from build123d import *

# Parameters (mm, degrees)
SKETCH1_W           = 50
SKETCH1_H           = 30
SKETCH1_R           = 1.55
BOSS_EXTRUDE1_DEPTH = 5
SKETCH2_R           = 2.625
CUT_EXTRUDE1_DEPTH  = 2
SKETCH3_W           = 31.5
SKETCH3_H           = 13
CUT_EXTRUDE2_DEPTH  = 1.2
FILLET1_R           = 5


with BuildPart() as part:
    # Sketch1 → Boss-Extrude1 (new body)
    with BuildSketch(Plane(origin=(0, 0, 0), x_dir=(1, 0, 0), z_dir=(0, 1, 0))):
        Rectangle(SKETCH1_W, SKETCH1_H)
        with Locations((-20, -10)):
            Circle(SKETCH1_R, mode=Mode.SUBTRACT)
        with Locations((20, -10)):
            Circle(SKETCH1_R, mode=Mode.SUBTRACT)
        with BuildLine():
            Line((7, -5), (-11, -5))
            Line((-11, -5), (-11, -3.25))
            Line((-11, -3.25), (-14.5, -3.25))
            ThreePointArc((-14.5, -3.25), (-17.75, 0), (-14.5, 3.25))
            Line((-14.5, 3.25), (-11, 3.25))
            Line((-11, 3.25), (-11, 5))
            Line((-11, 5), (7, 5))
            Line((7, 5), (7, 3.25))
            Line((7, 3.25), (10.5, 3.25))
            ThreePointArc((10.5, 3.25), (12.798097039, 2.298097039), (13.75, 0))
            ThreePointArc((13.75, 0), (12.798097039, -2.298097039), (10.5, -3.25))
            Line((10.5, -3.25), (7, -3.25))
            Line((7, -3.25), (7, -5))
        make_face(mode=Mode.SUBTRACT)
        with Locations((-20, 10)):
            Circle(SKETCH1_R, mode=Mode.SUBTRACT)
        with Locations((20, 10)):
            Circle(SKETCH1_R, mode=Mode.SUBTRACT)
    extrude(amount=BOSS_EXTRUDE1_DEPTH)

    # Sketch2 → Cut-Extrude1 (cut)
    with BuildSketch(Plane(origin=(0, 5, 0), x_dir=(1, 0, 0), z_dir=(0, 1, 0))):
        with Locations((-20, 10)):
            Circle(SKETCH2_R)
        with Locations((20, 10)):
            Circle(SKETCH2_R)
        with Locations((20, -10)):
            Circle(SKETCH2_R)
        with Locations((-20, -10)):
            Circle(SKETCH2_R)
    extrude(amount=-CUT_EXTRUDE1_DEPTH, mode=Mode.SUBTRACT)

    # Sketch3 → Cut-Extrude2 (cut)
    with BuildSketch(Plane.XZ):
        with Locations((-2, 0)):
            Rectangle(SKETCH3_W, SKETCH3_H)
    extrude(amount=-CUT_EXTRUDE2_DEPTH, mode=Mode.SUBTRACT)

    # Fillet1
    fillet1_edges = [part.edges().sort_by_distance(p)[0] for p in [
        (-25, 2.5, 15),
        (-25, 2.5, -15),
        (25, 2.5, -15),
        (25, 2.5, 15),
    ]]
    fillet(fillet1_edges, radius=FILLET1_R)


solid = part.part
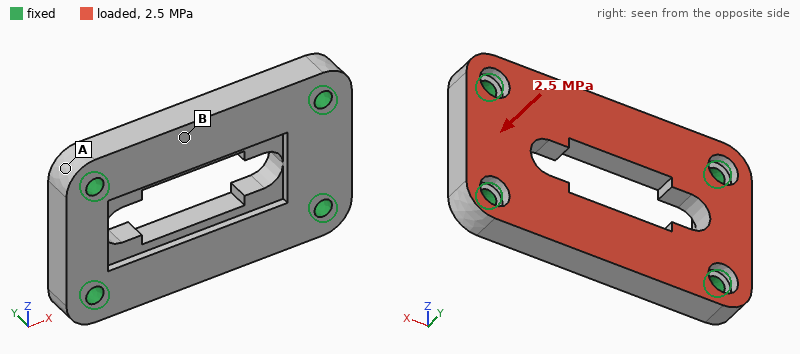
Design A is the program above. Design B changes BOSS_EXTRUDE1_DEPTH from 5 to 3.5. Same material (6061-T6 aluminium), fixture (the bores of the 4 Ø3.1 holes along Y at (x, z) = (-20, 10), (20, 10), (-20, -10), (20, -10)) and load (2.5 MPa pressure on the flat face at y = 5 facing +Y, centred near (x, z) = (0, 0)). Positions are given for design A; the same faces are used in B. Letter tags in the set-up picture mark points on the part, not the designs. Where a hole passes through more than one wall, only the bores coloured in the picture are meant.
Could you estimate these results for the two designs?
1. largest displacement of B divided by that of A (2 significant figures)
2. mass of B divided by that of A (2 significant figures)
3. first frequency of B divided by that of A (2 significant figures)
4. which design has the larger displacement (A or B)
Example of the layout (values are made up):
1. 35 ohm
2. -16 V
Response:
1. 2.1
2. 0.70
3. 0.86
4. B
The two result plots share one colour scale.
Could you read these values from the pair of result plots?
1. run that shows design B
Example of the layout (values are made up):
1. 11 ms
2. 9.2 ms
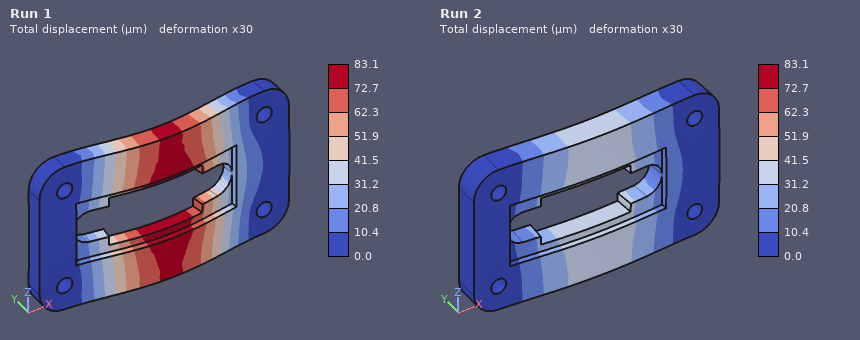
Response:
1. Run 1
